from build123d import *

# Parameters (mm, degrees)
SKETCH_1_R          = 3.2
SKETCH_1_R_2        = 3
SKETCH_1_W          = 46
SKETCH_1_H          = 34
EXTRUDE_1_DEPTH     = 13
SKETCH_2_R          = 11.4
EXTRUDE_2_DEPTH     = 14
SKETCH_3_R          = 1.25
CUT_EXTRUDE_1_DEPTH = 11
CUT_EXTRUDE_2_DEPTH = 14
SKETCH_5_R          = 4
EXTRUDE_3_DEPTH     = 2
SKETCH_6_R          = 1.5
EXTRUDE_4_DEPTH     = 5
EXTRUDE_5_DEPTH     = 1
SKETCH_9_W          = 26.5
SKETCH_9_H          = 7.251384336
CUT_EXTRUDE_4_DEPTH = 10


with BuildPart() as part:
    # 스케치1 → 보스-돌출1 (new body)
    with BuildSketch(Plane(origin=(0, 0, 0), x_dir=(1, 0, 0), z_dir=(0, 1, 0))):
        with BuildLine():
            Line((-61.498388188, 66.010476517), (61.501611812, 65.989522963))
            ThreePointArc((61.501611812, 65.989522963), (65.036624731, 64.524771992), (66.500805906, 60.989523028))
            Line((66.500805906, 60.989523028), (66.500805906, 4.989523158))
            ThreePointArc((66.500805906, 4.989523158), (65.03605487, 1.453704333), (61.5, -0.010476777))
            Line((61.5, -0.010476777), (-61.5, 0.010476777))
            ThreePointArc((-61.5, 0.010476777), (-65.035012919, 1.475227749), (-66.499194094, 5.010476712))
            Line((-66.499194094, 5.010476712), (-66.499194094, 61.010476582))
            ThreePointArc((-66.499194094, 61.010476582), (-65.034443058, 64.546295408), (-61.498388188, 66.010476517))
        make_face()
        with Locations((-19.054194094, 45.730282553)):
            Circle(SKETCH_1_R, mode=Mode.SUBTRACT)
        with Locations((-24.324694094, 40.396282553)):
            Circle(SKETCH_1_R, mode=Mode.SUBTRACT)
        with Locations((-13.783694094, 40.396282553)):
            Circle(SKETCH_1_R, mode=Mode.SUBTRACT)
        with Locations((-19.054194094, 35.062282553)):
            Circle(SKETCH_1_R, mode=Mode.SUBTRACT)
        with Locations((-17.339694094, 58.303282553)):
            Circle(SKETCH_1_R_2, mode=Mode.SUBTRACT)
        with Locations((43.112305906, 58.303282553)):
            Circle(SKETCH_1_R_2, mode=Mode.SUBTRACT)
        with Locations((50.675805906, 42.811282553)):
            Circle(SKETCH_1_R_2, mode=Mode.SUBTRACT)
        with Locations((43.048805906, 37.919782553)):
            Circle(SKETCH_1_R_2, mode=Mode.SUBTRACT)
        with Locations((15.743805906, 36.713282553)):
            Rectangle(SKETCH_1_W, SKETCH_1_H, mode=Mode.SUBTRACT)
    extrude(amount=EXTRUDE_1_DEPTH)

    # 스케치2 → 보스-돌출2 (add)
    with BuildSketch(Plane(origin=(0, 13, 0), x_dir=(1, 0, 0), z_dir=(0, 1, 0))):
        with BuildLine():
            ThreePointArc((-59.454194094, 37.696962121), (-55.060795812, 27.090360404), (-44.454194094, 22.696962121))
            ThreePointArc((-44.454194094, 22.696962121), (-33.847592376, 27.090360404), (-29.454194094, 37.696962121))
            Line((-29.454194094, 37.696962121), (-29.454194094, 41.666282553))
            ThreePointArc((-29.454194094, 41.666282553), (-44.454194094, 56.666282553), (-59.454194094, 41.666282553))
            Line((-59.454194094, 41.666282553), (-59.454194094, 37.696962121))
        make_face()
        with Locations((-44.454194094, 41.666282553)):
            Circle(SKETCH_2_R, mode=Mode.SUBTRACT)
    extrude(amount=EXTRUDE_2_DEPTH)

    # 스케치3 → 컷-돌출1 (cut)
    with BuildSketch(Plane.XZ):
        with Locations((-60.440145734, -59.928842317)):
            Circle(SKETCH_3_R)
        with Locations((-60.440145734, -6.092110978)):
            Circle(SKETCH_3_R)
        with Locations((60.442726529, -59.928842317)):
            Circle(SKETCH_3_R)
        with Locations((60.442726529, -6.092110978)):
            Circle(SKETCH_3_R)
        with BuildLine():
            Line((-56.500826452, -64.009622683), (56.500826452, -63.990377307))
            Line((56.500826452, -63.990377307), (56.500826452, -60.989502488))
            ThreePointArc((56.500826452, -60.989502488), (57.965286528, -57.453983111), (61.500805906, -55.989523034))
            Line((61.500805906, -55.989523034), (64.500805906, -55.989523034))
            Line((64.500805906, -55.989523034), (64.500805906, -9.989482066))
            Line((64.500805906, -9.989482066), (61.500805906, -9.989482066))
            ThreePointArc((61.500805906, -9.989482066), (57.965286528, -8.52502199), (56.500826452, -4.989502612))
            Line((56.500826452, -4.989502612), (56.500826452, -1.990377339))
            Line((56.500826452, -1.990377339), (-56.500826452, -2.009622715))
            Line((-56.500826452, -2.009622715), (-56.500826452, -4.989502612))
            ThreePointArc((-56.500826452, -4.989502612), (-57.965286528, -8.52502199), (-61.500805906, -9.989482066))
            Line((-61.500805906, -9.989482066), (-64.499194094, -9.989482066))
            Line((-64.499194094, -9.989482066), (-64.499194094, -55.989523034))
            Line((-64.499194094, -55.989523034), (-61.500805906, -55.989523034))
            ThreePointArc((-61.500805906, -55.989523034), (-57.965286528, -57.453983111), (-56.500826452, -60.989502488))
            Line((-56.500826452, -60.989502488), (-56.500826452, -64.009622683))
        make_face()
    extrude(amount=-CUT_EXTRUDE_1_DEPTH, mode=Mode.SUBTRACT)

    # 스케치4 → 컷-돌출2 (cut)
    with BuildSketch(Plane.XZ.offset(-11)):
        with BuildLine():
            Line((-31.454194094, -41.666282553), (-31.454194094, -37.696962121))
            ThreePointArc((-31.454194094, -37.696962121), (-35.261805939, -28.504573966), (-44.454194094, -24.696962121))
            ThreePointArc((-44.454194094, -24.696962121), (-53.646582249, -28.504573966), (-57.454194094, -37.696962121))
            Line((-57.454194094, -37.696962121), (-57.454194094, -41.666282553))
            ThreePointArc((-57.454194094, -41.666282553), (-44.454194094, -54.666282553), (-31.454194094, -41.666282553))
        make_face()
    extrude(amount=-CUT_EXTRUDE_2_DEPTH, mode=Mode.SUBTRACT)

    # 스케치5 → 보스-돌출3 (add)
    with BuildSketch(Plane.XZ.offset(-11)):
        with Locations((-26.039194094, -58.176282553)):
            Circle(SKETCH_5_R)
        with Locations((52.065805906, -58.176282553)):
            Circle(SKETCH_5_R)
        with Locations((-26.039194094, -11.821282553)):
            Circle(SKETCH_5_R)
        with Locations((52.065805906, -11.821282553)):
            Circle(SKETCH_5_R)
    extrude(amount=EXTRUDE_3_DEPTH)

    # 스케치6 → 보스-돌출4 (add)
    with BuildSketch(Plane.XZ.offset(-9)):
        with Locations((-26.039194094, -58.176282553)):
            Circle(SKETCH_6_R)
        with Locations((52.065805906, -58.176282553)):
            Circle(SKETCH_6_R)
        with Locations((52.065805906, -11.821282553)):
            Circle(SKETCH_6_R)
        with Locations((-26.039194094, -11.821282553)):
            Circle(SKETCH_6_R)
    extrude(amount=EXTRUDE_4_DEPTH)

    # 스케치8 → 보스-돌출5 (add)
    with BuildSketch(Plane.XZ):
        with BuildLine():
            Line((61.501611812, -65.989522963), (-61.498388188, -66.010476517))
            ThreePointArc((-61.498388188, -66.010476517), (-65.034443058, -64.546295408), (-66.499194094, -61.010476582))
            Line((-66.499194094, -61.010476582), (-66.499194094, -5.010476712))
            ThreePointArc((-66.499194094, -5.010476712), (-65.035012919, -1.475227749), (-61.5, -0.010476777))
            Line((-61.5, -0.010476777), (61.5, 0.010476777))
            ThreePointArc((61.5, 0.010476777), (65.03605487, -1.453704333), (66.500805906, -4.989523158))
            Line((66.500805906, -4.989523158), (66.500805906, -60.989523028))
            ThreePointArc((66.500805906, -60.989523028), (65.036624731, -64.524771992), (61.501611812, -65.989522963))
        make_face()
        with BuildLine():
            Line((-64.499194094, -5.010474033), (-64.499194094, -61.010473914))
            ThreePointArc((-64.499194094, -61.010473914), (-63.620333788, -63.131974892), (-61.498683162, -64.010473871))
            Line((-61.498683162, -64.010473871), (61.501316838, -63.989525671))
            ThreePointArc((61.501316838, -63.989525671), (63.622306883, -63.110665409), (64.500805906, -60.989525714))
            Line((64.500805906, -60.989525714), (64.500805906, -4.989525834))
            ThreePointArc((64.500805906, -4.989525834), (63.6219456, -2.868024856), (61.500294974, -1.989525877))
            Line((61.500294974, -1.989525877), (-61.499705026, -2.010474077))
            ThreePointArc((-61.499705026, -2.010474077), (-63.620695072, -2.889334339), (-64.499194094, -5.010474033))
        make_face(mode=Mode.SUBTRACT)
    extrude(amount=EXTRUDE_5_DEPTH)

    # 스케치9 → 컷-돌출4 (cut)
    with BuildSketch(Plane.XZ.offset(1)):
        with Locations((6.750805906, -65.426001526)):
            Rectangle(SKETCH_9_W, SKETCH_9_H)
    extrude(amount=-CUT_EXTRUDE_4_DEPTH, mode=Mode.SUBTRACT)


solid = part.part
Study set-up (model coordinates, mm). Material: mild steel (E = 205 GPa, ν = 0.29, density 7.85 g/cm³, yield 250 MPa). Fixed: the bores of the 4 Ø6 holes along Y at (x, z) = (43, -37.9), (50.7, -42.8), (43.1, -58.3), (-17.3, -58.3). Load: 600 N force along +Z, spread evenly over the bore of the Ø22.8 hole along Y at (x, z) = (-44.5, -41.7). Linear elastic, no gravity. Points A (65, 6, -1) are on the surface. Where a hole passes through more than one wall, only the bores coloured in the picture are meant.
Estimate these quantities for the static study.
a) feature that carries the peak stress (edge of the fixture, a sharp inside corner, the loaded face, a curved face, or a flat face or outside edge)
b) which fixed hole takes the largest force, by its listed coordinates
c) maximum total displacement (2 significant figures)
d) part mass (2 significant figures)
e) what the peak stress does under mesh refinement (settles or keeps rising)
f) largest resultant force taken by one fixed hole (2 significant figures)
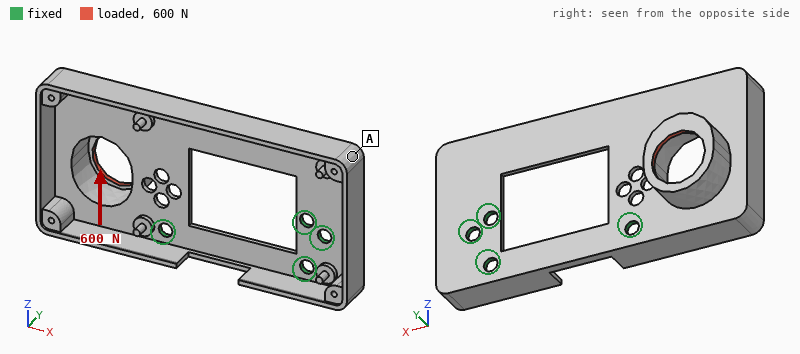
edge of the fixture
(-17.3, -58.3)
0.67 mm
210 g
keeps rising
670 N
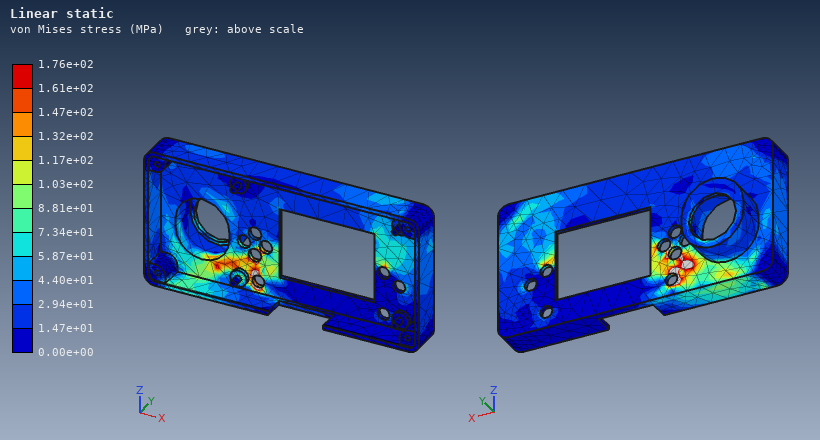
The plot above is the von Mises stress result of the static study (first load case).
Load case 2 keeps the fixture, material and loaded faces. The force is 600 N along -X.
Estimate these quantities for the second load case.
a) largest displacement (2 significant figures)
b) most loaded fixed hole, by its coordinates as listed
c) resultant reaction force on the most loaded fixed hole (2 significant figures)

0.34 mm
(-17.3, -58.3)
530 N
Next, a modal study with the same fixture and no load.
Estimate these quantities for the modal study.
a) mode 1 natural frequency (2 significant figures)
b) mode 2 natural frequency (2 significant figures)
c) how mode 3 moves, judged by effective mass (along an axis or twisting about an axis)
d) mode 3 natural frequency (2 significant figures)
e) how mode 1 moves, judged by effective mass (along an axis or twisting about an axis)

360 Hz
1000 Hz
along Y
1400 Hz
along Y
